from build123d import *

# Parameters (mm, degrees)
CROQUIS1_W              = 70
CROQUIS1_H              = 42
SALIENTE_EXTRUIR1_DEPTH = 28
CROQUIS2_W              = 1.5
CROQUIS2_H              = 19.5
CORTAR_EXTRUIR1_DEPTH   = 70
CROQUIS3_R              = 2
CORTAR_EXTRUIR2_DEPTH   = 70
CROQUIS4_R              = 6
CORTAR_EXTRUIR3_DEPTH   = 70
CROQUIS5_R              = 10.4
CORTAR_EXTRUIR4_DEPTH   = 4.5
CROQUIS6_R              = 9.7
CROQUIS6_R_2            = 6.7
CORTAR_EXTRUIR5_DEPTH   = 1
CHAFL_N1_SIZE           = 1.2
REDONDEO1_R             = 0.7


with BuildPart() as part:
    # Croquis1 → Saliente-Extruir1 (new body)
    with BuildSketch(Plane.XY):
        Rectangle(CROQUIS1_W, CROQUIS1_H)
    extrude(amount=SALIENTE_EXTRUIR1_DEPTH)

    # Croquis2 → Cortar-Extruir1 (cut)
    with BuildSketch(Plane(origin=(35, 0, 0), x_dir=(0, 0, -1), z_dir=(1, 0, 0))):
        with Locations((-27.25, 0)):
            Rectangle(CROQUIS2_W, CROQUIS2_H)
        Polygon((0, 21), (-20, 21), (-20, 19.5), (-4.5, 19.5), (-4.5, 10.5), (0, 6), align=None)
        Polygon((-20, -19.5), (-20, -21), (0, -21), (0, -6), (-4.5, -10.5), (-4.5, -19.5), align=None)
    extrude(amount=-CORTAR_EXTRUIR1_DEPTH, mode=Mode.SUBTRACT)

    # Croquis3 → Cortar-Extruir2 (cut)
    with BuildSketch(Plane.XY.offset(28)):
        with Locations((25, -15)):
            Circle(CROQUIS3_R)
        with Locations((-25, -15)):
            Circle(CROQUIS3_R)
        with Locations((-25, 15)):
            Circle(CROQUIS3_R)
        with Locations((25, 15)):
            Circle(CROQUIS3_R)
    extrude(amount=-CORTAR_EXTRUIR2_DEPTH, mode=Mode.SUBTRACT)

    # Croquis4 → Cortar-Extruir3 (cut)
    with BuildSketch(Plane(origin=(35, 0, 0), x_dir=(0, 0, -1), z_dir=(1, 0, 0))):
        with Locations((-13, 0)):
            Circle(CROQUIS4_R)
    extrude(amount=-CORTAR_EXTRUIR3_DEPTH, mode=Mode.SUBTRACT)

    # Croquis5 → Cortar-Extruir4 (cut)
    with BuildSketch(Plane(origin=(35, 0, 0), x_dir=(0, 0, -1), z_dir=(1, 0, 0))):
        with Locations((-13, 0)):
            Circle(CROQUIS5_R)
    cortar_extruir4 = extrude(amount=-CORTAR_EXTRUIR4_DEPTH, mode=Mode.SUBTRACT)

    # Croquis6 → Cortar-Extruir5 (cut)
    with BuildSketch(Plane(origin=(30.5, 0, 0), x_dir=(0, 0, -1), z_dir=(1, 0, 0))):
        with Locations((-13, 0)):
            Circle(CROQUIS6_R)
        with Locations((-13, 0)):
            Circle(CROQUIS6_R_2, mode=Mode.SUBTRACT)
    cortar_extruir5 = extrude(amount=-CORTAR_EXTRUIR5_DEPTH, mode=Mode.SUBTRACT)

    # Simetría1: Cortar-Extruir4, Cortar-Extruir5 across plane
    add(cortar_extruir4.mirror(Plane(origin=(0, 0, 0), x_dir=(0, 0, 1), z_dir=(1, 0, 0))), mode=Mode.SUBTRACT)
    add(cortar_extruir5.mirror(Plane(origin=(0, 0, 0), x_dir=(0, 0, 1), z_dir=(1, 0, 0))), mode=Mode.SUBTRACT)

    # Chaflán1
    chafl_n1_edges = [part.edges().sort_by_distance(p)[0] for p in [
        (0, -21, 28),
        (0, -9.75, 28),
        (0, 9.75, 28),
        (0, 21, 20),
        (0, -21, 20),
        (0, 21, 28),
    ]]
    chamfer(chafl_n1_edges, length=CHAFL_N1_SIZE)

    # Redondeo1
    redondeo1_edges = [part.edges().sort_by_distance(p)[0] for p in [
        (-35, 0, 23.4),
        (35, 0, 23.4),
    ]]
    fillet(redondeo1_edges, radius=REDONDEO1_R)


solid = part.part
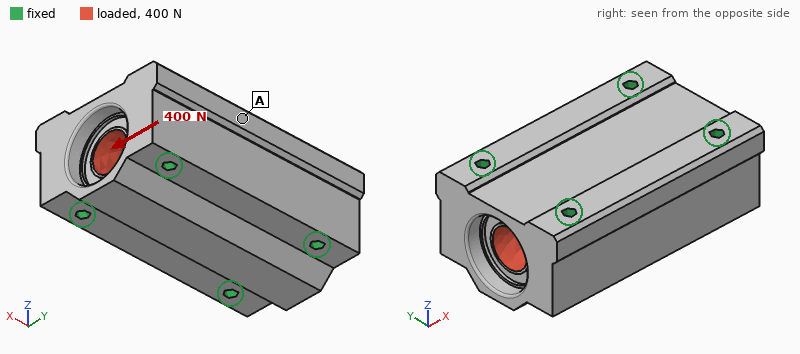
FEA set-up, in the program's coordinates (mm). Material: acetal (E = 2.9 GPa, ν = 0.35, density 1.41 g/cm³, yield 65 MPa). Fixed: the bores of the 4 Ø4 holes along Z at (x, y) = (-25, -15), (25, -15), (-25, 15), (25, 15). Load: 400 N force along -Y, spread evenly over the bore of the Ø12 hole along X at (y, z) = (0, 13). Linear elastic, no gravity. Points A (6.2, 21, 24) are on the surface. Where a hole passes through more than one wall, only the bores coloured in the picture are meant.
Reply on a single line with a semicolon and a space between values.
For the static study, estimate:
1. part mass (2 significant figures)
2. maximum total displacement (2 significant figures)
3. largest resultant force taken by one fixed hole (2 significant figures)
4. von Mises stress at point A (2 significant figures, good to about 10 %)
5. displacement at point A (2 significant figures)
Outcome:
81 g; 4.3 µm; 110 N; 0.19 MPa; 2.7 µm
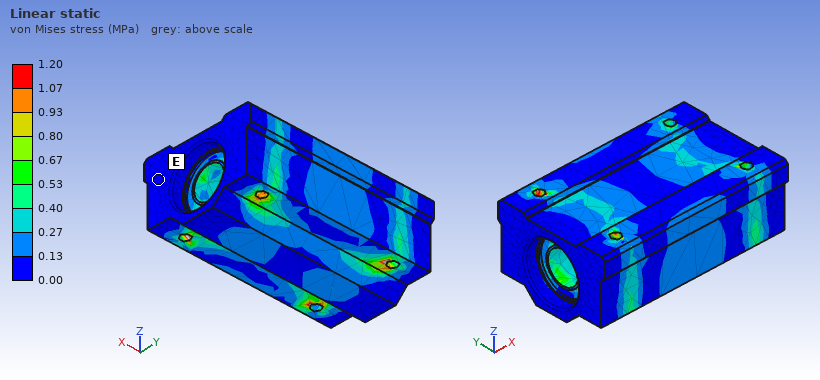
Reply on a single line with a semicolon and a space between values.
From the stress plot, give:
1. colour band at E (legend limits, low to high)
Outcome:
0.00 to 0.13 MPa
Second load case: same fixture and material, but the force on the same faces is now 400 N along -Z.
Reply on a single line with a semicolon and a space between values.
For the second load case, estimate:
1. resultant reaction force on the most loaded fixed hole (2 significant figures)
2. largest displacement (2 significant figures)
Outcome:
100 N; 5.7 µm
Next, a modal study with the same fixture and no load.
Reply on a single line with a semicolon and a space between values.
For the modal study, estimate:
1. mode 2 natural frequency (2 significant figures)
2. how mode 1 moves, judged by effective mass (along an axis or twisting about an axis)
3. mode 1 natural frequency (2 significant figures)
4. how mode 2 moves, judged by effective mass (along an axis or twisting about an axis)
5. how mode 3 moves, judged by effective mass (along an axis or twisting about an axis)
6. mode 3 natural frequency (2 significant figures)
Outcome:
7000 Hz; along Z; 6200 Hz; along Y; twisting about X; 7700 Hz
